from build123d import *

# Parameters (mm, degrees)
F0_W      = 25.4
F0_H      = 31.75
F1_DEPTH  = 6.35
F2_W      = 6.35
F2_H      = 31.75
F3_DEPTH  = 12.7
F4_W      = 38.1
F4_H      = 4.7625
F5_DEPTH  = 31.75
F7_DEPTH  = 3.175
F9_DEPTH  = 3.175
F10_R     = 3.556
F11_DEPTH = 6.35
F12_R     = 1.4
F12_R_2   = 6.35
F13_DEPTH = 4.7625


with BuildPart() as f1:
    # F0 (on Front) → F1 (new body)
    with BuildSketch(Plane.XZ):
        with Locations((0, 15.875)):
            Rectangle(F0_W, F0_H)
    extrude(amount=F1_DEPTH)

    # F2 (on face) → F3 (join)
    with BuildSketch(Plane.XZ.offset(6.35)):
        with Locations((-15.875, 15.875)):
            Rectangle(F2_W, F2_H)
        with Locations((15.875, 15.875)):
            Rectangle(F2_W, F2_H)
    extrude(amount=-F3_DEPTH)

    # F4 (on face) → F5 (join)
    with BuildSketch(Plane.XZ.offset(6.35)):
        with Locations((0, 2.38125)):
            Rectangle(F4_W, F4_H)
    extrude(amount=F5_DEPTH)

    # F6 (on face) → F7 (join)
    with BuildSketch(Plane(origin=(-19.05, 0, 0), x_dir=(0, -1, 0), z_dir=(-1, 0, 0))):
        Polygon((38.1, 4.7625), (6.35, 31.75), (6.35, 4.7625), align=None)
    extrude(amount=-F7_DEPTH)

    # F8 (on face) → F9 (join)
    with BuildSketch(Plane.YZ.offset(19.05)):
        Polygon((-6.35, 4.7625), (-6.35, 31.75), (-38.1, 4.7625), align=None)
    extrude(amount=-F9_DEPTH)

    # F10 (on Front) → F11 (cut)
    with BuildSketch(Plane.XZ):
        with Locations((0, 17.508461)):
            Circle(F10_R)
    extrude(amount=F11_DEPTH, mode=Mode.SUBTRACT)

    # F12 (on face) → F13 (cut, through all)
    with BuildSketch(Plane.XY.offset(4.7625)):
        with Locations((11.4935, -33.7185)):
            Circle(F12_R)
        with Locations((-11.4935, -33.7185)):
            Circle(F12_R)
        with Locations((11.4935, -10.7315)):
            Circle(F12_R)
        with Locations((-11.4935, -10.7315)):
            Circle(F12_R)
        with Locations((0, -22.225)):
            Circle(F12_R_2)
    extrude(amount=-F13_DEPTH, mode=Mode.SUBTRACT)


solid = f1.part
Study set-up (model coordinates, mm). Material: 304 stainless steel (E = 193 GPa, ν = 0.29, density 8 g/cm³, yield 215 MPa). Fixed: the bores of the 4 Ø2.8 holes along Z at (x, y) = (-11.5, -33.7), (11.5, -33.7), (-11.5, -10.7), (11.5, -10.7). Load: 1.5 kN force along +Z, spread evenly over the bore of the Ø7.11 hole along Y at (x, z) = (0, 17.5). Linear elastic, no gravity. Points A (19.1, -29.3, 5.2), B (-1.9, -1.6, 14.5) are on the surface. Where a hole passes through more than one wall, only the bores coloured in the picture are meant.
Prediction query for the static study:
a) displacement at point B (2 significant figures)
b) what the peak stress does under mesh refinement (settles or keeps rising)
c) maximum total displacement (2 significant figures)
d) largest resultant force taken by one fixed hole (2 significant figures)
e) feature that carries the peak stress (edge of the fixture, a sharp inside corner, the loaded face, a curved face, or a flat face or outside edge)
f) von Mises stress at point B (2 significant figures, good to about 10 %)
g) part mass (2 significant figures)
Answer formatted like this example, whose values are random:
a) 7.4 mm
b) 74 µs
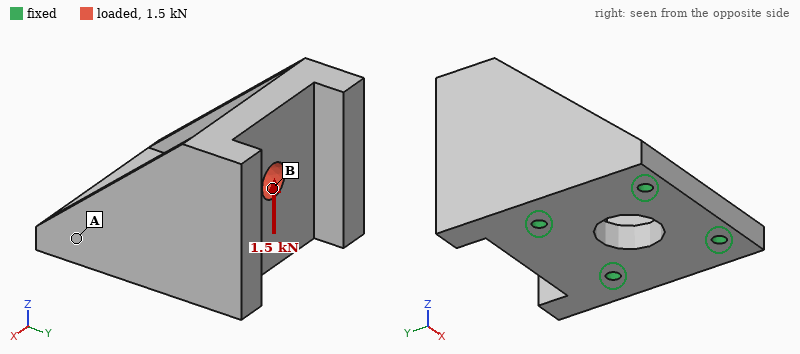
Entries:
a) 4.7 µm
b) keeps rising
c) 6.8 µm
d) 910 N
e) edge of the fixture
f) 14 MPa
g) 140 g
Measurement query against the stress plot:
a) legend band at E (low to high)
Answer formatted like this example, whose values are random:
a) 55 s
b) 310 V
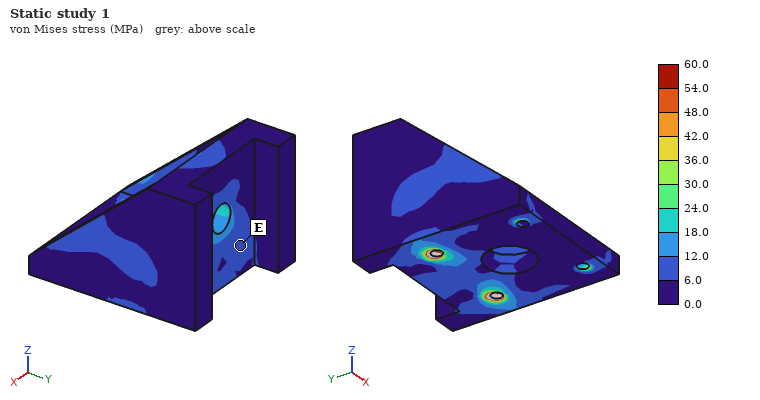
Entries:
a) 6.0 to 12.0 MPa
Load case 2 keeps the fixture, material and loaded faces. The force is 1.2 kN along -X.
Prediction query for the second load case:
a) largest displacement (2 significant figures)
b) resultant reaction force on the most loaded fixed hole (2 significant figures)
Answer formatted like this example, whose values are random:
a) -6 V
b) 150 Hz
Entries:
a) 8.2 µm
b) 980 N
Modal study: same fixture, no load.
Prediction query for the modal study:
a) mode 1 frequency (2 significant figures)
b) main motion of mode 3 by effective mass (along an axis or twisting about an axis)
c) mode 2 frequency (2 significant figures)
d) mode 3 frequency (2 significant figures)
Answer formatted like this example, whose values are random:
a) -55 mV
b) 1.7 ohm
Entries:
a) 6800 Hz
b) along X
c) 7000 Hz
d) 13 kHz
